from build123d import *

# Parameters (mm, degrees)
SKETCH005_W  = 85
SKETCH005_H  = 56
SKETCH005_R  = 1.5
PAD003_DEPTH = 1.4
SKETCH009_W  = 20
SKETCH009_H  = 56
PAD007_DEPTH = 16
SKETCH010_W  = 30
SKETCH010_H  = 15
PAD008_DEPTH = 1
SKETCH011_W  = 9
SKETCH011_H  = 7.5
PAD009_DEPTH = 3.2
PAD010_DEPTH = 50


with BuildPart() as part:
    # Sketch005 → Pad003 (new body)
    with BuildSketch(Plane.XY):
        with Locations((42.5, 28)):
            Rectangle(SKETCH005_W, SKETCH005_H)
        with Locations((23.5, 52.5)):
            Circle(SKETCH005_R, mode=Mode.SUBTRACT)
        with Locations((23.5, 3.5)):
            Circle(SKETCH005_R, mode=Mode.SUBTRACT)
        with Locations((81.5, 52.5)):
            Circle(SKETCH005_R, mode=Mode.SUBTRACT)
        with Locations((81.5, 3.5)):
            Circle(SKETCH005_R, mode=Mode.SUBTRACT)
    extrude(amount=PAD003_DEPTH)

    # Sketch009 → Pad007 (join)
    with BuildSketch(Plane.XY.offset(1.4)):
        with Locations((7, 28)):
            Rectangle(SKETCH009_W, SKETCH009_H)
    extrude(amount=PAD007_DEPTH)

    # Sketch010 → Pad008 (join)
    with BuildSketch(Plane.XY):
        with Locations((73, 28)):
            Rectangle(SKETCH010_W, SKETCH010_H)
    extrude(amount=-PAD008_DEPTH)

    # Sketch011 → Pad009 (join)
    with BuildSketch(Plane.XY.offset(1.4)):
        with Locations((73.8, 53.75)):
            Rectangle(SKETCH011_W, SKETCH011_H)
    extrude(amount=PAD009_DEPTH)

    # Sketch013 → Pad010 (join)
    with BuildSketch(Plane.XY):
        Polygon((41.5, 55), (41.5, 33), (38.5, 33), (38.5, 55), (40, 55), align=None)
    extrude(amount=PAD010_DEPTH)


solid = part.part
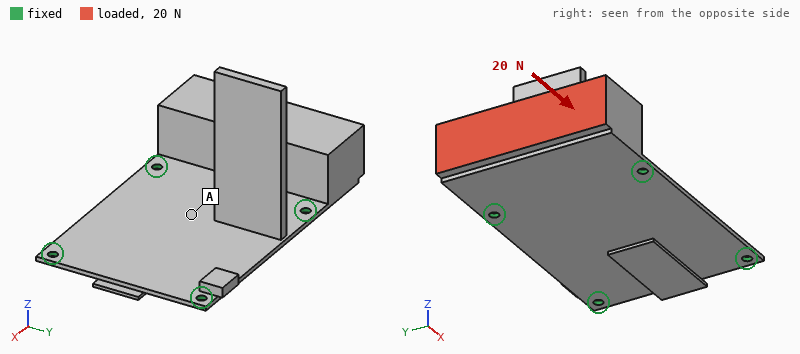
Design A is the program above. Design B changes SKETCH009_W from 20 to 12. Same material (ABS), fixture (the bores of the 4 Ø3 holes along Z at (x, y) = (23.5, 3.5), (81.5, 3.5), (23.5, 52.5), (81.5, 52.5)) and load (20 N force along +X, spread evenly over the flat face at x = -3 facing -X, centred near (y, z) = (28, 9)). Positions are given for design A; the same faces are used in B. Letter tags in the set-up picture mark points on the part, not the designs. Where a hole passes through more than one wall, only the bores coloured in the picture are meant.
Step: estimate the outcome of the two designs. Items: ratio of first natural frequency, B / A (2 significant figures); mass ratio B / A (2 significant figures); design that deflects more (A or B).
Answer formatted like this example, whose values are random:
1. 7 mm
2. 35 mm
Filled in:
1. 1.2
2. 0.75
3. B
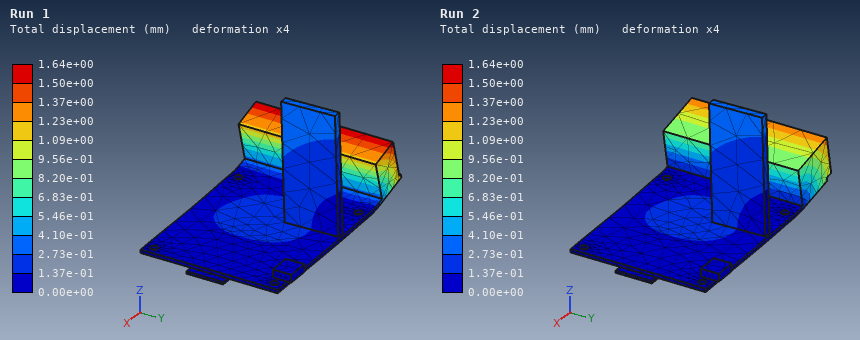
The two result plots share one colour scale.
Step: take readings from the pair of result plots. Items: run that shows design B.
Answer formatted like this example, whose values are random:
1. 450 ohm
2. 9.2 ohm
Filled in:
1. Run 1
